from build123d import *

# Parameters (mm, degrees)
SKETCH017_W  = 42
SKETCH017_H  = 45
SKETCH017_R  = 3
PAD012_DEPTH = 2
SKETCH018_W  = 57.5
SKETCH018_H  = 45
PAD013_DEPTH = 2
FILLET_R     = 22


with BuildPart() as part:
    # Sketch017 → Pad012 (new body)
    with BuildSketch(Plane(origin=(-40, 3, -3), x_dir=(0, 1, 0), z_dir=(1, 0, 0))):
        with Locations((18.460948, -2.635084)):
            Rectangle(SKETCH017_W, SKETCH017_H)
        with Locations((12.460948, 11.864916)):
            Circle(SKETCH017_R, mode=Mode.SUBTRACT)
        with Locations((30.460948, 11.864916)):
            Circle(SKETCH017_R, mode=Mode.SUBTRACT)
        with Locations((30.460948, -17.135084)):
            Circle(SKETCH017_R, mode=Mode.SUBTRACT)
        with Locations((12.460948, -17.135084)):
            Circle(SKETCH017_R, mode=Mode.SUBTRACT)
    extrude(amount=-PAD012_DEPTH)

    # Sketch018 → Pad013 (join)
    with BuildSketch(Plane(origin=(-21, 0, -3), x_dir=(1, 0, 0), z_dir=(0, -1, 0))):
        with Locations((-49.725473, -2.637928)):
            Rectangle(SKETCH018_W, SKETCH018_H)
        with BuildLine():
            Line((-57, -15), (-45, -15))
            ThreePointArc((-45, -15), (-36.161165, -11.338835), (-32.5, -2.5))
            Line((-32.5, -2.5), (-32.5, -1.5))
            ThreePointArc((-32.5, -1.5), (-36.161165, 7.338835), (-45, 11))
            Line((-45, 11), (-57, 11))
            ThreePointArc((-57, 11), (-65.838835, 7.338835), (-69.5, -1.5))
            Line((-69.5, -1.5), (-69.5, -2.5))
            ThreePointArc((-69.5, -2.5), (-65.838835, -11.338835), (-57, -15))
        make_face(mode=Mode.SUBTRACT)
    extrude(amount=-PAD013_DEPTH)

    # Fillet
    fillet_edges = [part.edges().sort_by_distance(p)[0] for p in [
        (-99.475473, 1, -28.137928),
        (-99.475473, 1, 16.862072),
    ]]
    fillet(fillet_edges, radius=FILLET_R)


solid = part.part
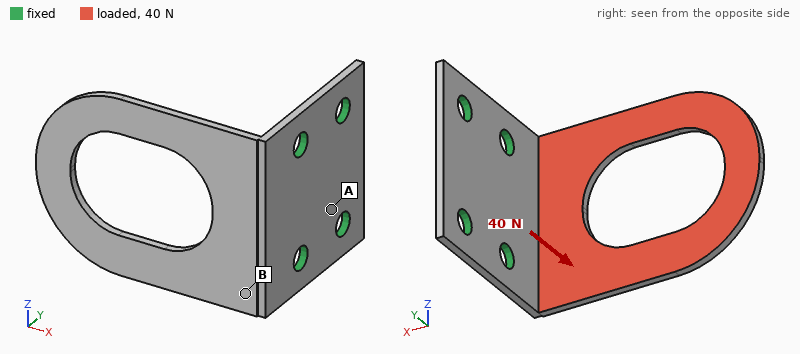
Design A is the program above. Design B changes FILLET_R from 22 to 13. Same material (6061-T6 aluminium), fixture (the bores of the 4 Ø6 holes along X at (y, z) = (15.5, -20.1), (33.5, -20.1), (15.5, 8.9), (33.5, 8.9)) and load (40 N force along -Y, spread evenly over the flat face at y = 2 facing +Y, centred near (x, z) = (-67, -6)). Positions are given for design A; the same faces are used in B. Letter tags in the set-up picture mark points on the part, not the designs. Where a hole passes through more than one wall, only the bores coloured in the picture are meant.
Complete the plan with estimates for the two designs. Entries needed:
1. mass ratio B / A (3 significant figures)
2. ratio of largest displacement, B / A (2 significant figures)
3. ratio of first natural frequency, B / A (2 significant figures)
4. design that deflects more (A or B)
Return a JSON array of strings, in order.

["1.04", "1.1", "0.88", "B"]
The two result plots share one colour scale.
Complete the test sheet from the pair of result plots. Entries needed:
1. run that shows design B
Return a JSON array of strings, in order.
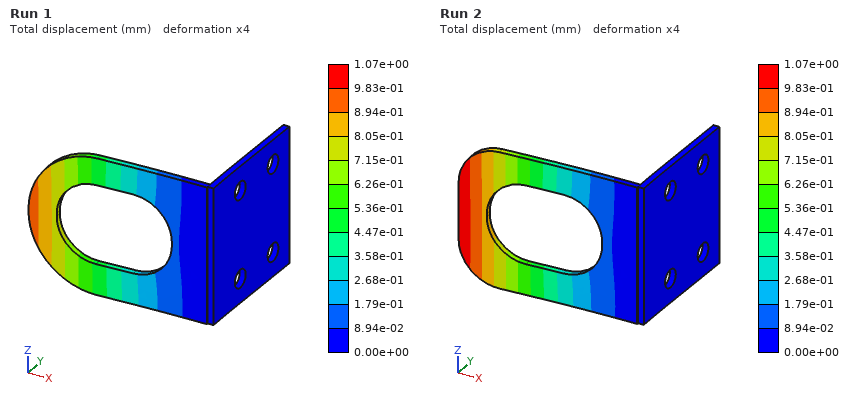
["Run 2"]
